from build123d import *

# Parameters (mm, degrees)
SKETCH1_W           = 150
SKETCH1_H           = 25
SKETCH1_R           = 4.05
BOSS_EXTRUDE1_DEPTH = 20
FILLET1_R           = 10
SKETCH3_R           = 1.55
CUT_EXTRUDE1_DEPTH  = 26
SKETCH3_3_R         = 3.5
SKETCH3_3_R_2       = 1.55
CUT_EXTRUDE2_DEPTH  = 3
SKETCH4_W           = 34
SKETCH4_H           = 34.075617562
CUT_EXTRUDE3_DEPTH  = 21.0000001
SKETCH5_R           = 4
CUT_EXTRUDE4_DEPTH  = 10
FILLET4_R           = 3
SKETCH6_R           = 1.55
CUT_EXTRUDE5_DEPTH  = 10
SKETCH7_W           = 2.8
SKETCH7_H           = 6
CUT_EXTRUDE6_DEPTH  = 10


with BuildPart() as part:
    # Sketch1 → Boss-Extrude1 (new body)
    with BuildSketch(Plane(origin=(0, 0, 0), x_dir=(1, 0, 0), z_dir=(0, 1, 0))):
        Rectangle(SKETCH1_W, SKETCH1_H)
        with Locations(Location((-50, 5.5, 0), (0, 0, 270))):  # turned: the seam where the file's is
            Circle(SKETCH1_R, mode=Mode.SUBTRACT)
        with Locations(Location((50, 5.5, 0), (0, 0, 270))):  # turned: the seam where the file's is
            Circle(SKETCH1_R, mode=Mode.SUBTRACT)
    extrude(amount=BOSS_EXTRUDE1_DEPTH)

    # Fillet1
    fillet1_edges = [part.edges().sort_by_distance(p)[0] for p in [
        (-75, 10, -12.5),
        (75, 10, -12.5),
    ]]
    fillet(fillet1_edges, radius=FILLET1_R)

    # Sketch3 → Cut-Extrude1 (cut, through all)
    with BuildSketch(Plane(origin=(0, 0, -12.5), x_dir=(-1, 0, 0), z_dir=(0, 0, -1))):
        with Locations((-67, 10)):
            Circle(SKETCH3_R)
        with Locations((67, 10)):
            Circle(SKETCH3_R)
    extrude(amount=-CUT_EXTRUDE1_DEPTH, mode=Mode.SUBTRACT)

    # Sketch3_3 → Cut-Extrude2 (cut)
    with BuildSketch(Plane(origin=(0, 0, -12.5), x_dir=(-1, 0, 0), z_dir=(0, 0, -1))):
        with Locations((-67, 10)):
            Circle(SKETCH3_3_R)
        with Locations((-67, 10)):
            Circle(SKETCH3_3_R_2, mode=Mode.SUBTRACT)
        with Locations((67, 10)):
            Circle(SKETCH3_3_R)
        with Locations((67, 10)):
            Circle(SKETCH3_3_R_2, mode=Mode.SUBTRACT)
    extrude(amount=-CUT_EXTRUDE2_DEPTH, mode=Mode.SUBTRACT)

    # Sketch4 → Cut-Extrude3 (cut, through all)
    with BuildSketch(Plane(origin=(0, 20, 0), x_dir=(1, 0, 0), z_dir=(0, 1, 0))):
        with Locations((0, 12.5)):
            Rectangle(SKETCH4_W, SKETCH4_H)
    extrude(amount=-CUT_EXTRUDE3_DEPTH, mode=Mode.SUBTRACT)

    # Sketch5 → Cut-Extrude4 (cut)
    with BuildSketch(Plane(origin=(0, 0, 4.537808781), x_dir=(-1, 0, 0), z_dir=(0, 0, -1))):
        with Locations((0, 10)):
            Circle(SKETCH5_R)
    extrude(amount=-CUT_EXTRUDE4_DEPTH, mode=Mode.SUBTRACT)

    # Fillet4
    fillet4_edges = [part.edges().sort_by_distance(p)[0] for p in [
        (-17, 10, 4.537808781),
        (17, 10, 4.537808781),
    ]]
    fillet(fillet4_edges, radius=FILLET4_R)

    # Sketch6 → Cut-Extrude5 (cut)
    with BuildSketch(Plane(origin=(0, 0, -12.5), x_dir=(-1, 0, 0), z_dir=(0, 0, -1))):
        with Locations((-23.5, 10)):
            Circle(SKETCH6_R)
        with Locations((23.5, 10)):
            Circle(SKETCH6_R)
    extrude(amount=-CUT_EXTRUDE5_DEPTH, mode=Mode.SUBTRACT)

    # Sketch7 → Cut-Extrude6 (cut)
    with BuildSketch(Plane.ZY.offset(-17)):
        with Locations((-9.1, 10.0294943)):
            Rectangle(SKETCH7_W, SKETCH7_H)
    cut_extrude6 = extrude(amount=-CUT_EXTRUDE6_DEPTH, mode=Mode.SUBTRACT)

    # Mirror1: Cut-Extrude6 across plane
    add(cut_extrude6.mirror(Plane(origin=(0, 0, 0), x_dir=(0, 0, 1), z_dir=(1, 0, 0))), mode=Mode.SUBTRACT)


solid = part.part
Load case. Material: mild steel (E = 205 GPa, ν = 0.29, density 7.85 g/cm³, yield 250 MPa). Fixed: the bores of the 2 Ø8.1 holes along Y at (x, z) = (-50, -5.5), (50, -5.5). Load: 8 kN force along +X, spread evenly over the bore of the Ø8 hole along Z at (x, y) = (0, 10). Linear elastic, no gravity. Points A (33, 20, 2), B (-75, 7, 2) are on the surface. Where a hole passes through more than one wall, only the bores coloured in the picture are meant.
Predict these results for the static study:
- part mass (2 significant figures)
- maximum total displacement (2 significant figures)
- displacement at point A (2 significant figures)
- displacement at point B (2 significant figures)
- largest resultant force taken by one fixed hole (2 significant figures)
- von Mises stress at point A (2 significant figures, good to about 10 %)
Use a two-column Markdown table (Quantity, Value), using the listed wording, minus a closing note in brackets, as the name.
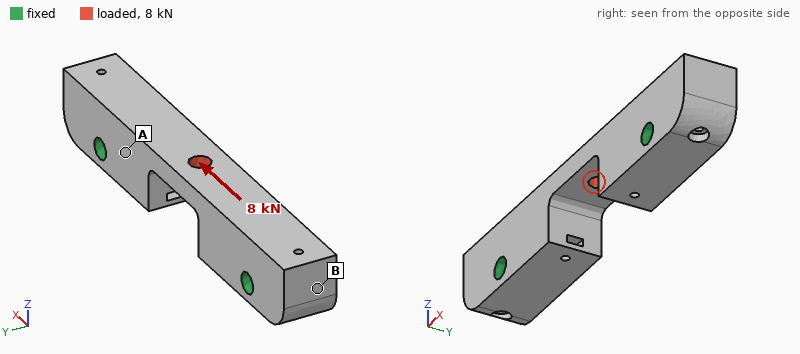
| Quantity | Value |
|---|---|
| part mass | 460 g |
| maximum total displacement | 7.4 µm |
| displacement at point A | 2.3 µm |
| displacement at point B | 2.5 µm |
| largest resultant force taken by one fixed hole | 4.0 kN |
| von Mises stress at point A | 12 MPa |
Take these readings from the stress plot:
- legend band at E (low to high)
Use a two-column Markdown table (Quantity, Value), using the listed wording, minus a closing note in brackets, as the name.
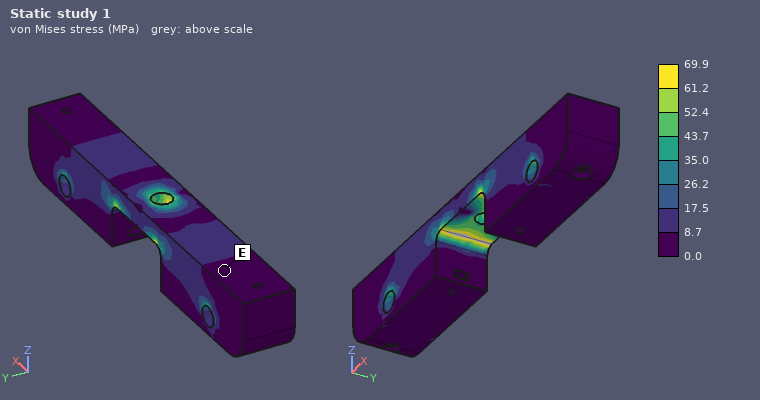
| Quantity | Value |
|---|---|
| legend band at E | 0.0 to 8.7 MPa |
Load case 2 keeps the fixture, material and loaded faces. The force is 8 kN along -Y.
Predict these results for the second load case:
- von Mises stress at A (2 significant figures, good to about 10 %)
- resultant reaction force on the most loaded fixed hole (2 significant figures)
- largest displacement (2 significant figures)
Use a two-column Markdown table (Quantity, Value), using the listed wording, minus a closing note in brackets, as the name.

| Quantity | Value |
|---|---|
| von Mises stress at A | 49 MPa |
| resultant reaction force on the most loaded fixed hole | 4.0 kN |
| largest displacement | 37 µm |
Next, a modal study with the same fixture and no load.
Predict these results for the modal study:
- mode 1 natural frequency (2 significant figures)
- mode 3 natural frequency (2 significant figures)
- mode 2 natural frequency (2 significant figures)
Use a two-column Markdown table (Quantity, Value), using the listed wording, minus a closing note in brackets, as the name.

| Quantity | Value |
|---|---|
| mode 1 natural frequency | 9800 Hz |
| mode 3 natural frequency | 11 kHz |
| mode 2 natural frequency | 9800 Hz |
